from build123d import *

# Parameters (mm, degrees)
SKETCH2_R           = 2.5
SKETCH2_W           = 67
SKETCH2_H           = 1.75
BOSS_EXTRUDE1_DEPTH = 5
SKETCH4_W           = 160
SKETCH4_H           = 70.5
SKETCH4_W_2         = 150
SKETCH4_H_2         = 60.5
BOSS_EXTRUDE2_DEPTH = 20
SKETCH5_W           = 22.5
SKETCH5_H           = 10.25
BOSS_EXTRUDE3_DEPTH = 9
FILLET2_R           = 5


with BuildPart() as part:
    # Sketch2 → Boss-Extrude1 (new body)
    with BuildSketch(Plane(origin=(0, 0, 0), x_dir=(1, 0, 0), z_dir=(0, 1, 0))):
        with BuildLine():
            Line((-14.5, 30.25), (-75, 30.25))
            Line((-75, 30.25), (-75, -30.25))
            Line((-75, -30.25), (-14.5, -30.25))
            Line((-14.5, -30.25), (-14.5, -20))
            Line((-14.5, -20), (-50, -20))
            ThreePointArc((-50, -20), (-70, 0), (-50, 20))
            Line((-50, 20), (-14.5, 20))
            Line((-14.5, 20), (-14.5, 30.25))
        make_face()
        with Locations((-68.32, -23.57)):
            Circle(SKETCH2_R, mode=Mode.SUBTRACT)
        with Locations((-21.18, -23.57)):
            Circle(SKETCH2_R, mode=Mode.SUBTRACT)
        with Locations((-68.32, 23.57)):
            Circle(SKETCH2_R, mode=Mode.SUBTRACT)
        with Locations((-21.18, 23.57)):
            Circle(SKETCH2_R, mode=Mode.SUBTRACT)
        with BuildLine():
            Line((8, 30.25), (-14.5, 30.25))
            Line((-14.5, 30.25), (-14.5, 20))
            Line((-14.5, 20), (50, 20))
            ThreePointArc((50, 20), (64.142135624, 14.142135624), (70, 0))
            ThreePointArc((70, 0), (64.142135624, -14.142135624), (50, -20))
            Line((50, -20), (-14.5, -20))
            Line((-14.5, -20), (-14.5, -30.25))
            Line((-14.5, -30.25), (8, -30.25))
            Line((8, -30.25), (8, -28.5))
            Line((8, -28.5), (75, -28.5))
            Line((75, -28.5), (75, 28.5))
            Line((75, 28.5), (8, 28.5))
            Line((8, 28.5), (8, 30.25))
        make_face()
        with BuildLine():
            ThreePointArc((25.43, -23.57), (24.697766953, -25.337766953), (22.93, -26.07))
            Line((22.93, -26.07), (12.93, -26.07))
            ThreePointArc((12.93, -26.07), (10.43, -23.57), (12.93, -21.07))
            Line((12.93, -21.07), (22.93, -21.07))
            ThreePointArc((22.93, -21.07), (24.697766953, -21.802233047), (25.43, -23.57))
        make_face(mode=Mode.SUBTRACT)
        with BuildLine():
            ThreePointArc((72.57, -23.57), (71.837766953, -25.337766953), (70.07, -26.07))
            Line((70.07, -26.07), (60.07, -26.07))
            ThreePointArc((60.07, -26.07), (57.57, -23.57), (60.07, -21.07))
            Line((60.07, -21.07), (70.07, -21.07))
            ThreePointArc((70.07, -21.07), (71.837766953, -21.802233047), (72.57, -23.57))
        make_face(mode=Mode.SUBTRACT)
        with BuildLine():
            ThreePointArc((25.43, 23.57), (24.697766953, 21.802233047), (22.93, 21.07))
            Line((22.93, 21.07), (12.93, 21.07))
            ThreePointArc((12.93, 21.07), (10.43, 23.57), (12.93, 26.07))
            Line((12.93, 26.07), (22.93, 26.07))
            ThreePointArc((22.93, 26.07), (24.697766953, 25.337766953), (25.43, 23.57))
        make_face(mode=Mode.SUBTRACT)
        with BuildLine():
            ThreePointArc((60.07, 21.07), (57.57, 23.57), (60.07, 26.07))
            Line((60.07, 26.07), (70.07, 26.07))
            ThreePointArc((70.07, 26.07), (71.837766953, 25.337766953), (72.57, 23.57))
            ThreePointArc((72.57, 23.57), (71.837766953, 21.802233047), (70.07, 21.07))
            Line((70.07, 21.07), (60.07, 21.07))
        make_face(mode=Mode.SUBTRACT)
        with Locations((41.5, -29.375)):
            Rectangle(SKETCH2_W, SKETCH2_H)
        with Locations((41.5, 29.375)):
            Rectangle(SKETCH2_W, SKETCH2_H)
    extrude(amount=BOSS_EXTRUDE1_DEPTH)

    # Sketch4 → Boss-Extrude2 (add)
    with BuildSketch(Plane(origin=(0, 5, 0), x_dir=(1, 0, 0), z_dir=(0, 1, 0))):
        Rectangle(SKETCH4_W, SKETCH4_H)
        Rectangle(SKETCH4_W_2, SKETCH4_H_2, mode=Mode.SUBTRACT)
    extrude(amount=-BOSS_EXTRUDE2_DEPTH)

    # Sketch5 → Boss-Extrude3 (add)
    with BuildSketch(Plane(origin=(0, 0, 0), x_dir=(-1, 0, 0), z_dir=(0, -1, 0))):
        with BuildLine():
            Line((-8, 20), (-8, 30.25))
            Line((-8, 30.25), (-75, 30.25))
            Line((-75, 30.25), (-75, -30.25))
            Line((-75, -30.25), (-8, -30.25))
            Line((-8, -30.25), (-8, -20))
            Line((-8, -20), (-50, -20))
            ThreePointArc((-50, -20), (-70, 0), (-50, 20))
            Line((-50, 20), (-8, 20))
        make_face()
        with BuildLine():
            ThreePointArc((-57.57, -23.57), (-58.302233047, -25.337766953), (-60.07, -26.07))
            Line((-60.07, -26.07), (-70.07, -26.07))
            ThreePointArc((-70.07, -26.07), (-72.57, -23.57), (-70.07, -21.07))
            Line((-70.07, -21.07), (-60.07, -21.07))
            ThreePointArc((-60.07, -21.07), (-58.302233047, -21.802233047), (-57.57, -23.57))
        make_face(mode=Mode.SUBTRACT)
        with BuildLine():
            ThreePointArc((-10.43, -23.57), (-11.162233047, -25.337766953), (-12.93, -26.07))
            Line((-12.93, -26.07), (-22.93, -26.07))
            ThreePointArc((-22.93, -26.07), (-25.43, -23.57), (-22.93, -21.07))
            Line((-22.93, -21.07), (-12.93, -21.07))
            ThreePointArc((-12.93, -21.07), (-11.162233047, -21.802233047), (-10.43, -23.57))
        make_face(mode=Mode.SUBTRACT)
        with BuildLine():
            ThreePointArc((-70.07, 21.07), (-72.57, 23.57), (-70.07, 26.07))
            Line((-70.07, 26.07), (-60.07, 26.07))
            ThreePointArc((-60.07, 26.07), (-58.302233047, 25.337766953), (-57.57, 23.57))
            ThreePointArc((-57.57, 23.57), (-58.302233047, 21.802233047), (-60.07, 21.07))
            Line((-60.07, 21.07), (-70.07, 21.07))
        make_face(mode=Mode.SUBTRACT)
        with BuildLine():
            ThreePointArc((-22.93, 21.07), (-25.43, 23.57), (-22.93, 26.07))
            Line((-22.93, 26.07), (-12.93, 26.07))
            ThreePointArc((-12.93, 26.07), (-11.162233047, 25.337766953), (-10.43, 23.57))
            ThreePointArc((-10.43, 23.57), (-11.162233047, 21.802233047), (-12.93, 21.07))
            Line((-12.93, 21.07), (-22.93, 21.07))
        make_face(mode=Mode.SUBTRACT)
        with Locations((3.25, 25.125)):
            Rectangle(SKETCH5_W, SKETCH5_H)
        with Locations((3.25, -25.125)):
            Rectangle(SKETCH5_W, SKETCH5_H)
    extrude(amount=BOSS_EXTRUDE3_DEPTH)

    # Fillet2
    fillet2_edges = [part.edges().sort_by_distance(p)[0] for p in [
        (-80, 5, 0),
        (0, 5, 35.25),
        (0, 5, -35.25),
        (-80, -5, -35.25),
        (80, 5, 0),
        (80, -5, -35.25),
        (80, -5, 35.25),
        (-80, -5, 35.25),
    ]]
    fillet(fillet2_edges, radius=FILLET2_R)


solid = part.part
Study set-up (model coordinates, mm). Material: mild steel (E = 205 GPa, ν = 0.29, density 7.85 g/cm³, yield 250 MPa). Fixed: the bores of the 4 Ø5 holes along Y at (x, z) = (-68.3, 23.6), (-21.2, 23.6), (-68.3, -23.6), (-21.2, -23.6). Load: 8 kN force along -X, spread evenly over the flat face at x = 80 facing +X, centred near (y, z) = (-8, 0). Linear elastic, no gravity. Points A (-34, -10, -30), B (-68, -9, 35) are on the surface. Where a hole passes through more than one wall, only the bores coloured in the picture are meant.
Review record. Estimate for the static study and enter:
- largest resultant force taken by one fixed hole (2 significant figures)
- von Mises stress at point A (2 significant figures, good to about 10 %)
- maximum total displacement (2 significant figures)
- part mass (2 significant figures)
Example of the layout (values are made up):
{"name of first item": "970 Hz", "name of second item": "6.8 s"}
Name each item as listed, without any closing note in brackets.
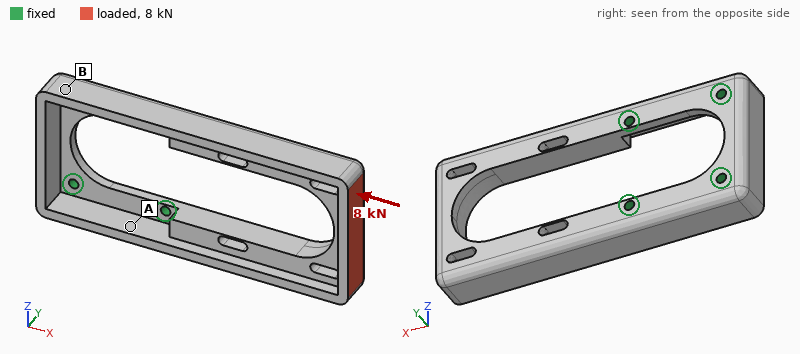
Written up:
{"largest resultant force taken by one fixed hole": "2.5 kN", "von Mises stress at point A": "32 MPa", "maximum total displacement": "0.15 mm", "part mass": "600 g"}
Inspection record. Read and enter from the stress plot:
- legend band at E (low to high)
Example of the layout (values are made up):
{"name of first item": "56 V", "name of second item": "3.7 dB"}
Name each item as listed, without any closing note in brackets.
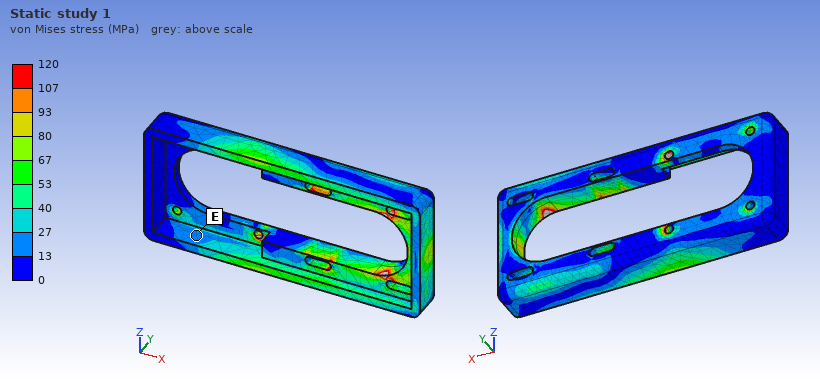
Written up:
{"legend band at E": "13 to 27 MPa"}
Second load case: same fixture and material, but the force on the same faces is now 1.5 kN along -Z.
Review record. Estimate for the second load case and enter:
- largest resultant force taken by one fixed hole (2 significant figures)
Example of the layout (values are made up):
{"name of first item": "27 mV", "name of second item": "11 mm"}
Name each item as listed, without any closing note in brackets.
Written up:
{"largest resultant force taken by one fixed hole": "1.4 kN"}
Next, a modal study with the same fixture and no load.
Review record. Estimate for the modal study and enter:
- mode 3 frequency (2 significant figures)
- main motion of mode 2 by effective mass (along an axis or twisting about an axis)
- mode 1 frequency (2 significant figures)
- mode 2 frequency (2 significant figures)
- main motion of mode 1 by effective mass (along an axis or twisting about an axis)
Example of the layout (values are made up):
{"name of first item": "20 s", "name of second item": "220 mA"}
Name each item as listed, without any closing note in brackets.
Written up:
{"mode 3 frequency": "1700 Hz", "main motion of mode 2 by effective mass": "along Z", "mode 1 frequency": "830 Hz", "mode 2 frequency": "1200 Hz", "main motion of mode 1 by effective mass": "along Y"}
